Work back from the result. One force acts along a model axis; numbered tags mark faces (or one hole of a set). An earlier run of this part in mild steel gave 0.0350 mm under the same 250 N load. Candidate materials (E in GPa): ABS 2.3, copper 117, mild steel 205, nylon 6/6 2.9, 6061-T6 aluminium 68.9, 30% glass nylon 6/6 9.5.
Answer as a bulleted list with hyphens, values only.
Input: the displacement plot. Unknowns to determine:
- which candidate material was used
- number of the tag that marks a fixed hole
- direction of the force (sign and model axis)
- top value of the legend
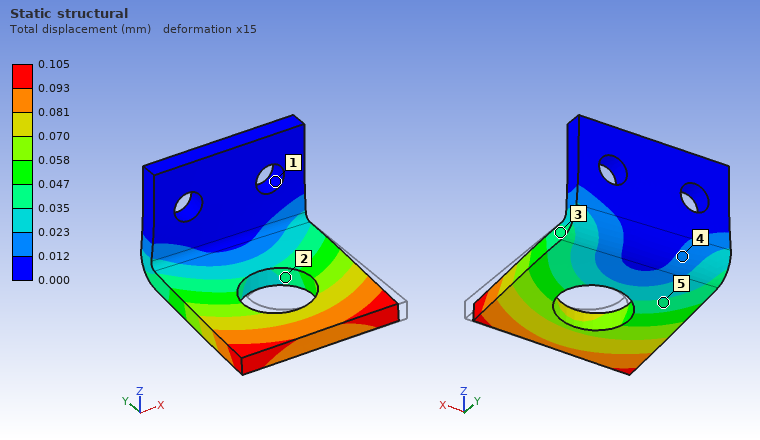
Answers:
- 6061-T6 aluminium
- 1
- -X
- 0.105 mm
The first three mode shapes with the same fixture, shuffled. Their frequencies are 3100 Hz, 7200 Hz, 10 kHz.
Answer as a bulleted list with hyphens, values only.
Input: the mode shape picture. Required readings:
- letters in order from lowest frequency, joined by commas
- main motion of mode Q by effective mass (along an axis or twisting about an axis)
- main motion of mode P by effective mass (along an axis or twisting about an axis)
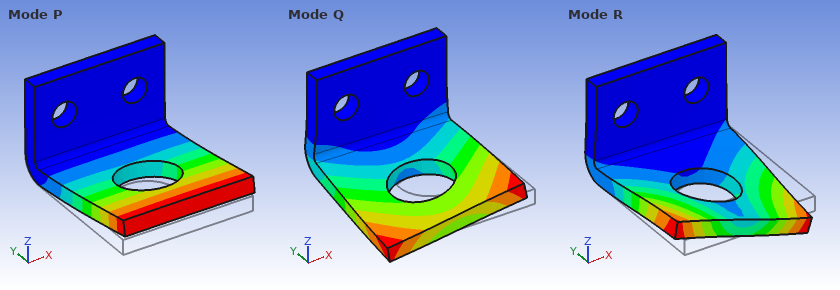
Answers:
- P, Q, R
- along X
- along Z
